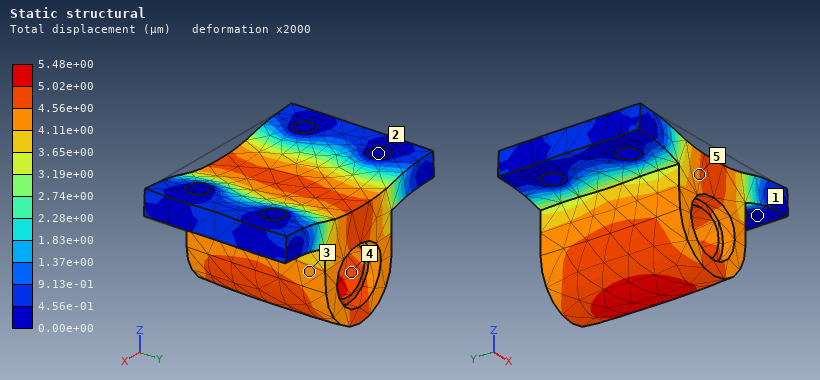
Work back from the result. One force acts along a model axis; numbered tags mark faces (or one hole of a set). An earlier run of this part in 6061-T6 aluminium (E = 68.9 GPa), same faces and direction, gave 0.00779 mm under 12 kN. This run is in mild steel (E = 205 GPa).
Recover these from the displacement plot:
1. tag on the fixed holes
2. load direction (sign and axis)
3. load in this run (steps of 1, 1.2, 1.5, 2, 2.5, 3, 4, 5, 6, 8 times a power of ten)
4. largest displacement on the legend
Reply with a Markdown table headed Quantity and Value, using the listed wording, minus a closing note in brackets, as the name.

| Quantity | Value |
|---|---|
| tag on the fixed holes | 2 |
| load direction | -Z |
| load in this run | 25 kN |
| largest displacement on the legend | 5.48e+00 µm |
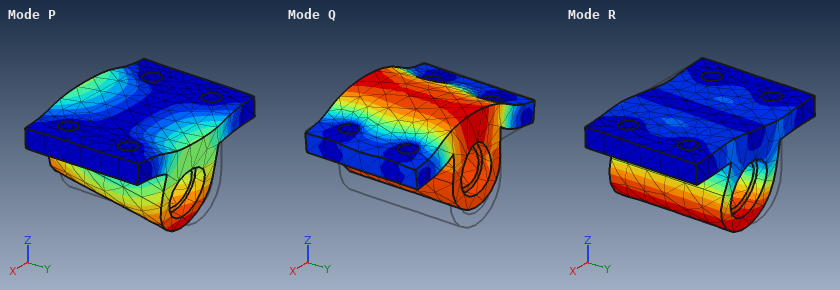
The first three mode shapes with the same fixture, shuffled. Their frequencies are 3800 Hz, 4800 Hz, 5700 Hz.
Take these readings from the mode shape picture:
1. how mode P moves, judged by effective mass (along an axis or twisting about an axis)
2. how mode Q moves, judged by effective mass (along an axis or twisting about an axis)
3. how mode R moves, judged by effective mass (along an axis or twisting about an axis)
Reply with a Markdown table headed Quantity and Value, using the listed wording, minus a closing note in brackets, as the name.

| Quantity | Value |
|---|---|
| how mode P moves, judged by effective mass | along Y |
| how mode Q moves, judged by effective mass | along Z |
| how mode R moves, judged by effective mass | along X |
